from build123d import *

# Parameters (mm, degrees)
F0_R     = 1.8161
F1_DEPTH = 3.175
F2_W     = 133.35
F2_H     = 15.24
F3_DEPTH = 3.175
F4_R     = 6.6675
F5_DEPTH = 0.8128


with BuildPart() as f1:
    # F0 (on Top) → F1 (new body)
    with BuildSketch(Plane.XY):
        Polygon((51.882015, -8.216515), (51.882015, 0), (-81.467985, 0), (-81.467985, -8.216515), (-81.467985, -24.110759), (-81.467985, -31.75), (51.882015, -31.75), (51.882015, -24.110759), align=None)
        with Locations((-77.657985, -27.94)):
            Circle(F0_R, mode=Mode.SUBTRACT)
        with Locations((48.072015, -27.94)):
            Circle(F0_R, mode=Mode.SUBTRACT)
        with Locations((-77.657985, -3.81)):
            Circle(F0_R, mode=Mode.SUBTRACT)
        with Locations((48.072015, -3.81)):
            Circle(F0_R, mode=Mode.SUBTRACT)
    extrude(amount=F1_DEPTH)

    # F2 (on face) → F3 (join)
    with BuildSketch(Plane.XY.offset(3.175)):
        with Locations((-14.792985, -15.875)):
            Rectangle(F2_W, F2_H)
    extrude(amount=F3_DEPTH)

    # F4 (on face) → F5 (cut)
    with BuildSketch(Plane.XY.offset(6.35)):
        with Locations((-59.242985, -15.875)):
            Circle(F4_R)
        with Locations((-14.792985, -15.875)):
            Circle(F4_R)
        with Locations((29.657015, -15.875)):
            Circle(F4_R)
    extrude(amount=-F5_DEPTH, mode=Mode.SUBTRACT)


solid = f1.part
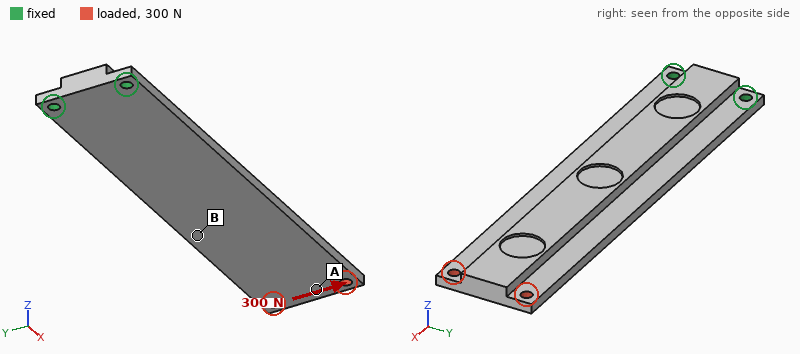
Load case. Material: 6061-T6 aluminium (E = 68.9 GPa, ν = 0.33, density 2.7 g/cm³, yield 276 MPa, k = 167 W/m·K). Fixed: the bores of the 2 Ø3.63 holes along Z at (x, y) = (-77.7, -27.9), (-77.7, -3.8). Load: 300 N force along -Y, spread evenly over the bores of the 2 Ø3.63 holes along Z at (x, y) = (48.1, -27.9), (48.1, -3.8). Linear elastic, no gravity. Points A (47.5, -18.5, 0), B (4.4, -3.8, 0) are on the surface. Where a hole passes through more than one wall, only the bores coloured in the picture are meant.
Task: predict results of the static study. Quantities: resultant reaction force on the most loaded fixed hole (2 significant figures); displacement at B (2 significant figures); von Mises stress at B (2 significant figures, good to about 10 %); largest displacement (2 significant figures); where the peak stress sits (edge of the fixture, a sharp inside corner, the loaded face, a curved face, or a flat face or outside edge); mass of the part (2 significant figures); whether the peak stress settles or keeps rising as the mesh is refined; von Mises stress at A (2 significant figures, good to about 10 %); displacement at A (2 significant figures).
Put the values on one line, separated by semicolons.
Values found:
1.5 kN; 0.17 mm; 18 MPa; 0.35 mm; edge of the fixture; 52 g; keeps rising; 5.8 MPa; 0.33 mm
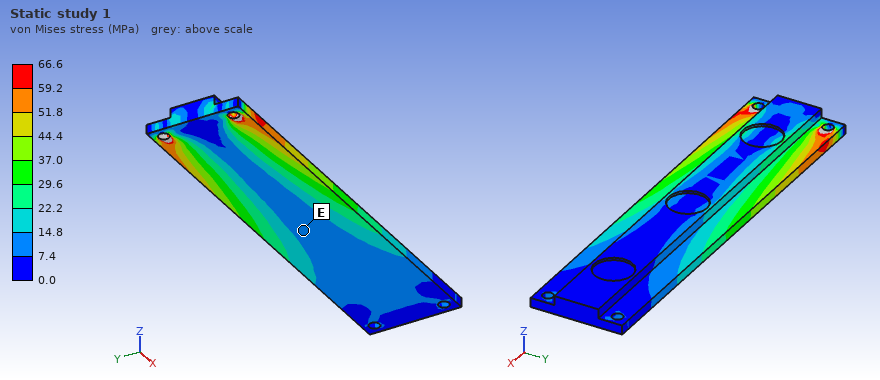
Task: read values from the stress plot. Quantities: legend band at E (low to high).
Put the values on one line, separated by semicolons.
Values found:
7.4 to 14.8 MPa
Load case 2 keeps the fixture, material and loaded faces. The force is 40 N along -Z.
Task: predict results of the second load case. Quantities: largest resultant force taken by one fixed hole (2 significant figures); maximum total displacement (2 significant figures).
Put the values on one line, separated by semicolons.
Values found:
42 N; 1.4 mm
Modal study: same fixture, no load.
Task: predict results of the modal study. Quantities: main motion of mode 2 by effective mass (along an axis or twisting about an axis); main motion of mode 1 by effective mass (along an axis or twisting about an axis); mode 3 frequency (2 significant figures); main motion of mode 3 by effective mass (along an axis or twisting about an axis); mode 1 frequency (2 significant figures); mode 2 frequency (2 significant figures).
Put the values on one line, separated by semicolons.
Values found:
along Y; along Z; 1500 Hz; along Z; 230 Hz; 1300 Hz
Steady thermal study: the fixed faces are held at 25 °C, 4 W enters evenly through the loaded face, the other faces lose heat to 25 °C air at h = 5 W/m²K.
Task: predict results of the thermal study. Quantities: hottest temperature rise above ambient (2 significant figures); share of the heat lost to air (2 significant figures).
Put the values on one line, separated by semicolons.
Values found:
21 K; 13 %
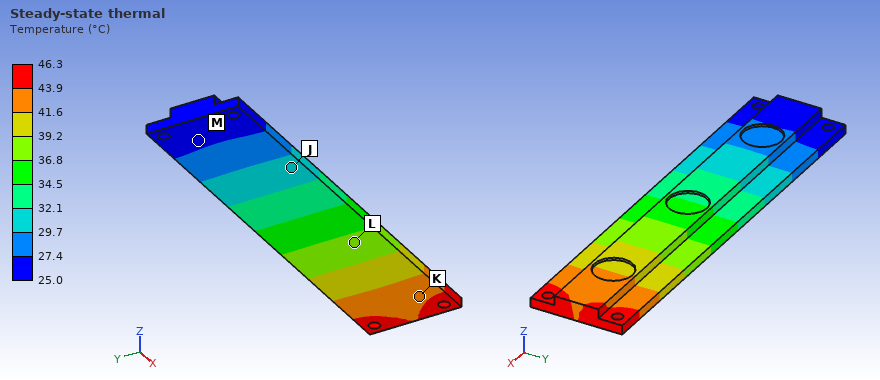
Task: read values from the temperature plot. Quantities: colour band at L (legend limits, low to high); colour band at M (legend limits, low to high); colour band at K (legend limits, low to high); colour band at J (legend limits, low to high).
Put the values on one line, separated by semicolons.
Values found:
36.8 to 39.2 °C; 25.0 to 27.4 °C; 41.6 to 43.9 °C; 29.7 to 32.1 °C
